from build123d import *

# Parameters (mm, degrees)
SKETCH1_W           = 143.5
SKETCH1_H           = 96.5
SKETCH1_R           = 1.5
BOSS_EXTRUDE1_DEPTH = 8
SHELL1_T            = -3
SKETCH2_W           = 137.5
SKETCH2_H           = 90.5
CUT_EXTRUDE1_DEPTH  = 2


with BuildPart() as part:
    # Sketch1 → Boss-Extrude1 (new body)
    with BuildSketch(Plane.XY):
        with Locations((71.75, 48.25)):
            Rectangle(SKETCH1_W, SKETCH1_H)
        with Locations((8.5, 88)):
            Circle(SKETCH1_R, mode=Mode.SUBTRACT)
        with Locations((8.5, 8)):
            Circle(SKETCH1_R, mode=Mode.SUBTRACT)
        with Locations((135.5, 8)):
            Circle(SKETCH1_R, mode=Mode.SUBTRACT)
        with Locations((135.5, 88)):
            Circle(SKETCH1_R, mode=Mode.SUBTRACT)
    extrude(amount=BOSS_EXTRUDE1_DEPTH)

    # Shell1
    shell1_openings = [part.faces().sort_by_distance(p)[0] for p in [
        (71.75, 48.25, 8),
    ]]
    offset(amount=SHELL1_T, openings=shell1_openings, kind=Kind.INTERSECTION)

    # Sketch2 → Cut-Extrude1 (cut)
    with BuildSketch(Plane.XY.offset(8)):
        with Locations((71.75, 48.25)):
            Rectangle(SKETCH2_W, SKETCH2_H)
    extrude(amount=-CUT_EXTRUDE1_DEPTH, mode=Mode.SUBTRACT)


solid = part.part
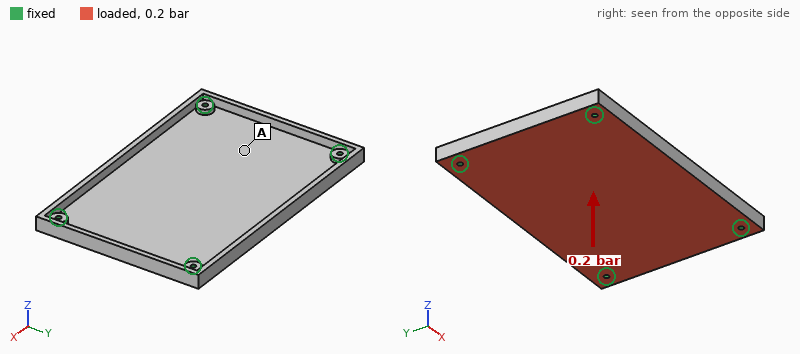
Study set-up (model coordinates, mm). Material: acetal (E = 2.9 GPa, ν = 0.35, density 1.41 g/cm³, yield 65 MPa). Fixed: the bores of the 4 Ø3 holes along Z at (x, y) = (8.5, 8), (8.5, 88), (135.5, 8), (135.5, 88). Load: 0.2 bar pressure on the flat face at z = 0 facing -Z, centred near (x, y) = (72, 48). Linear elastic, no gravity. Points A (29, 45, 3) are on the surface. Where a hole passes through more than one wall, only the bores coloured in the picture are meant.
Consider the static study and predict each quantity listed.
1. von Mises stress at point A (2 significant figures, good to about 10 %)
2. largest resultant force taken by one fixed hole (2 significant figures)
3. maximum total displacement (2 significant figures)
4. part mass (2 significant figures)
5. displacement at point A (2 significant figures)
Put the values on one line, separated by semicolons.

4.0 MPa; 74 N; 1.7 mm; 69 g; 0.87 mm
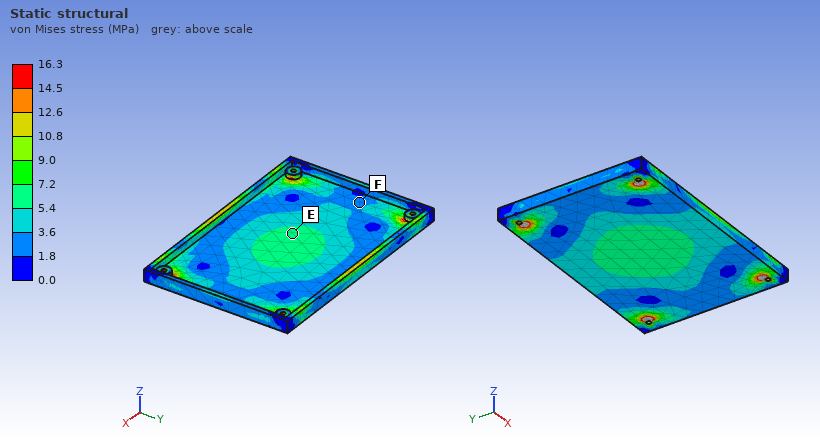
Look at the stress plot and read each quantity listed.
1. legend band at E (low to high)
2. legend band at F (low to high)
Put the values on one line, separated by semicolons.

5.4 to 7.2 MPa; 1.8 to 3.6 MPa
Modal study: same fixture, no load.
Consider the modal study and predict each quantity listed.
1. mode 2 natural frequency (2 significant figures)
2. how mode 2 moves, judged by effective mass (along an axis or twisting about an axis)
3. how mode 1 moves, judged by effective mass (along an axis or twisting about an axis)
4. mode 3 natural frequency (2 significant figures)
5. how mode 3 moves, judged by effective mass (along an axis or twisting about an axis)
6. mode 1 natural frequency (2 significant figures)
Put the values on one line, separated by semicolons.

520 Hz; twisting about X; along Z; 710 Hz; twisting about Y; 320 Hz
